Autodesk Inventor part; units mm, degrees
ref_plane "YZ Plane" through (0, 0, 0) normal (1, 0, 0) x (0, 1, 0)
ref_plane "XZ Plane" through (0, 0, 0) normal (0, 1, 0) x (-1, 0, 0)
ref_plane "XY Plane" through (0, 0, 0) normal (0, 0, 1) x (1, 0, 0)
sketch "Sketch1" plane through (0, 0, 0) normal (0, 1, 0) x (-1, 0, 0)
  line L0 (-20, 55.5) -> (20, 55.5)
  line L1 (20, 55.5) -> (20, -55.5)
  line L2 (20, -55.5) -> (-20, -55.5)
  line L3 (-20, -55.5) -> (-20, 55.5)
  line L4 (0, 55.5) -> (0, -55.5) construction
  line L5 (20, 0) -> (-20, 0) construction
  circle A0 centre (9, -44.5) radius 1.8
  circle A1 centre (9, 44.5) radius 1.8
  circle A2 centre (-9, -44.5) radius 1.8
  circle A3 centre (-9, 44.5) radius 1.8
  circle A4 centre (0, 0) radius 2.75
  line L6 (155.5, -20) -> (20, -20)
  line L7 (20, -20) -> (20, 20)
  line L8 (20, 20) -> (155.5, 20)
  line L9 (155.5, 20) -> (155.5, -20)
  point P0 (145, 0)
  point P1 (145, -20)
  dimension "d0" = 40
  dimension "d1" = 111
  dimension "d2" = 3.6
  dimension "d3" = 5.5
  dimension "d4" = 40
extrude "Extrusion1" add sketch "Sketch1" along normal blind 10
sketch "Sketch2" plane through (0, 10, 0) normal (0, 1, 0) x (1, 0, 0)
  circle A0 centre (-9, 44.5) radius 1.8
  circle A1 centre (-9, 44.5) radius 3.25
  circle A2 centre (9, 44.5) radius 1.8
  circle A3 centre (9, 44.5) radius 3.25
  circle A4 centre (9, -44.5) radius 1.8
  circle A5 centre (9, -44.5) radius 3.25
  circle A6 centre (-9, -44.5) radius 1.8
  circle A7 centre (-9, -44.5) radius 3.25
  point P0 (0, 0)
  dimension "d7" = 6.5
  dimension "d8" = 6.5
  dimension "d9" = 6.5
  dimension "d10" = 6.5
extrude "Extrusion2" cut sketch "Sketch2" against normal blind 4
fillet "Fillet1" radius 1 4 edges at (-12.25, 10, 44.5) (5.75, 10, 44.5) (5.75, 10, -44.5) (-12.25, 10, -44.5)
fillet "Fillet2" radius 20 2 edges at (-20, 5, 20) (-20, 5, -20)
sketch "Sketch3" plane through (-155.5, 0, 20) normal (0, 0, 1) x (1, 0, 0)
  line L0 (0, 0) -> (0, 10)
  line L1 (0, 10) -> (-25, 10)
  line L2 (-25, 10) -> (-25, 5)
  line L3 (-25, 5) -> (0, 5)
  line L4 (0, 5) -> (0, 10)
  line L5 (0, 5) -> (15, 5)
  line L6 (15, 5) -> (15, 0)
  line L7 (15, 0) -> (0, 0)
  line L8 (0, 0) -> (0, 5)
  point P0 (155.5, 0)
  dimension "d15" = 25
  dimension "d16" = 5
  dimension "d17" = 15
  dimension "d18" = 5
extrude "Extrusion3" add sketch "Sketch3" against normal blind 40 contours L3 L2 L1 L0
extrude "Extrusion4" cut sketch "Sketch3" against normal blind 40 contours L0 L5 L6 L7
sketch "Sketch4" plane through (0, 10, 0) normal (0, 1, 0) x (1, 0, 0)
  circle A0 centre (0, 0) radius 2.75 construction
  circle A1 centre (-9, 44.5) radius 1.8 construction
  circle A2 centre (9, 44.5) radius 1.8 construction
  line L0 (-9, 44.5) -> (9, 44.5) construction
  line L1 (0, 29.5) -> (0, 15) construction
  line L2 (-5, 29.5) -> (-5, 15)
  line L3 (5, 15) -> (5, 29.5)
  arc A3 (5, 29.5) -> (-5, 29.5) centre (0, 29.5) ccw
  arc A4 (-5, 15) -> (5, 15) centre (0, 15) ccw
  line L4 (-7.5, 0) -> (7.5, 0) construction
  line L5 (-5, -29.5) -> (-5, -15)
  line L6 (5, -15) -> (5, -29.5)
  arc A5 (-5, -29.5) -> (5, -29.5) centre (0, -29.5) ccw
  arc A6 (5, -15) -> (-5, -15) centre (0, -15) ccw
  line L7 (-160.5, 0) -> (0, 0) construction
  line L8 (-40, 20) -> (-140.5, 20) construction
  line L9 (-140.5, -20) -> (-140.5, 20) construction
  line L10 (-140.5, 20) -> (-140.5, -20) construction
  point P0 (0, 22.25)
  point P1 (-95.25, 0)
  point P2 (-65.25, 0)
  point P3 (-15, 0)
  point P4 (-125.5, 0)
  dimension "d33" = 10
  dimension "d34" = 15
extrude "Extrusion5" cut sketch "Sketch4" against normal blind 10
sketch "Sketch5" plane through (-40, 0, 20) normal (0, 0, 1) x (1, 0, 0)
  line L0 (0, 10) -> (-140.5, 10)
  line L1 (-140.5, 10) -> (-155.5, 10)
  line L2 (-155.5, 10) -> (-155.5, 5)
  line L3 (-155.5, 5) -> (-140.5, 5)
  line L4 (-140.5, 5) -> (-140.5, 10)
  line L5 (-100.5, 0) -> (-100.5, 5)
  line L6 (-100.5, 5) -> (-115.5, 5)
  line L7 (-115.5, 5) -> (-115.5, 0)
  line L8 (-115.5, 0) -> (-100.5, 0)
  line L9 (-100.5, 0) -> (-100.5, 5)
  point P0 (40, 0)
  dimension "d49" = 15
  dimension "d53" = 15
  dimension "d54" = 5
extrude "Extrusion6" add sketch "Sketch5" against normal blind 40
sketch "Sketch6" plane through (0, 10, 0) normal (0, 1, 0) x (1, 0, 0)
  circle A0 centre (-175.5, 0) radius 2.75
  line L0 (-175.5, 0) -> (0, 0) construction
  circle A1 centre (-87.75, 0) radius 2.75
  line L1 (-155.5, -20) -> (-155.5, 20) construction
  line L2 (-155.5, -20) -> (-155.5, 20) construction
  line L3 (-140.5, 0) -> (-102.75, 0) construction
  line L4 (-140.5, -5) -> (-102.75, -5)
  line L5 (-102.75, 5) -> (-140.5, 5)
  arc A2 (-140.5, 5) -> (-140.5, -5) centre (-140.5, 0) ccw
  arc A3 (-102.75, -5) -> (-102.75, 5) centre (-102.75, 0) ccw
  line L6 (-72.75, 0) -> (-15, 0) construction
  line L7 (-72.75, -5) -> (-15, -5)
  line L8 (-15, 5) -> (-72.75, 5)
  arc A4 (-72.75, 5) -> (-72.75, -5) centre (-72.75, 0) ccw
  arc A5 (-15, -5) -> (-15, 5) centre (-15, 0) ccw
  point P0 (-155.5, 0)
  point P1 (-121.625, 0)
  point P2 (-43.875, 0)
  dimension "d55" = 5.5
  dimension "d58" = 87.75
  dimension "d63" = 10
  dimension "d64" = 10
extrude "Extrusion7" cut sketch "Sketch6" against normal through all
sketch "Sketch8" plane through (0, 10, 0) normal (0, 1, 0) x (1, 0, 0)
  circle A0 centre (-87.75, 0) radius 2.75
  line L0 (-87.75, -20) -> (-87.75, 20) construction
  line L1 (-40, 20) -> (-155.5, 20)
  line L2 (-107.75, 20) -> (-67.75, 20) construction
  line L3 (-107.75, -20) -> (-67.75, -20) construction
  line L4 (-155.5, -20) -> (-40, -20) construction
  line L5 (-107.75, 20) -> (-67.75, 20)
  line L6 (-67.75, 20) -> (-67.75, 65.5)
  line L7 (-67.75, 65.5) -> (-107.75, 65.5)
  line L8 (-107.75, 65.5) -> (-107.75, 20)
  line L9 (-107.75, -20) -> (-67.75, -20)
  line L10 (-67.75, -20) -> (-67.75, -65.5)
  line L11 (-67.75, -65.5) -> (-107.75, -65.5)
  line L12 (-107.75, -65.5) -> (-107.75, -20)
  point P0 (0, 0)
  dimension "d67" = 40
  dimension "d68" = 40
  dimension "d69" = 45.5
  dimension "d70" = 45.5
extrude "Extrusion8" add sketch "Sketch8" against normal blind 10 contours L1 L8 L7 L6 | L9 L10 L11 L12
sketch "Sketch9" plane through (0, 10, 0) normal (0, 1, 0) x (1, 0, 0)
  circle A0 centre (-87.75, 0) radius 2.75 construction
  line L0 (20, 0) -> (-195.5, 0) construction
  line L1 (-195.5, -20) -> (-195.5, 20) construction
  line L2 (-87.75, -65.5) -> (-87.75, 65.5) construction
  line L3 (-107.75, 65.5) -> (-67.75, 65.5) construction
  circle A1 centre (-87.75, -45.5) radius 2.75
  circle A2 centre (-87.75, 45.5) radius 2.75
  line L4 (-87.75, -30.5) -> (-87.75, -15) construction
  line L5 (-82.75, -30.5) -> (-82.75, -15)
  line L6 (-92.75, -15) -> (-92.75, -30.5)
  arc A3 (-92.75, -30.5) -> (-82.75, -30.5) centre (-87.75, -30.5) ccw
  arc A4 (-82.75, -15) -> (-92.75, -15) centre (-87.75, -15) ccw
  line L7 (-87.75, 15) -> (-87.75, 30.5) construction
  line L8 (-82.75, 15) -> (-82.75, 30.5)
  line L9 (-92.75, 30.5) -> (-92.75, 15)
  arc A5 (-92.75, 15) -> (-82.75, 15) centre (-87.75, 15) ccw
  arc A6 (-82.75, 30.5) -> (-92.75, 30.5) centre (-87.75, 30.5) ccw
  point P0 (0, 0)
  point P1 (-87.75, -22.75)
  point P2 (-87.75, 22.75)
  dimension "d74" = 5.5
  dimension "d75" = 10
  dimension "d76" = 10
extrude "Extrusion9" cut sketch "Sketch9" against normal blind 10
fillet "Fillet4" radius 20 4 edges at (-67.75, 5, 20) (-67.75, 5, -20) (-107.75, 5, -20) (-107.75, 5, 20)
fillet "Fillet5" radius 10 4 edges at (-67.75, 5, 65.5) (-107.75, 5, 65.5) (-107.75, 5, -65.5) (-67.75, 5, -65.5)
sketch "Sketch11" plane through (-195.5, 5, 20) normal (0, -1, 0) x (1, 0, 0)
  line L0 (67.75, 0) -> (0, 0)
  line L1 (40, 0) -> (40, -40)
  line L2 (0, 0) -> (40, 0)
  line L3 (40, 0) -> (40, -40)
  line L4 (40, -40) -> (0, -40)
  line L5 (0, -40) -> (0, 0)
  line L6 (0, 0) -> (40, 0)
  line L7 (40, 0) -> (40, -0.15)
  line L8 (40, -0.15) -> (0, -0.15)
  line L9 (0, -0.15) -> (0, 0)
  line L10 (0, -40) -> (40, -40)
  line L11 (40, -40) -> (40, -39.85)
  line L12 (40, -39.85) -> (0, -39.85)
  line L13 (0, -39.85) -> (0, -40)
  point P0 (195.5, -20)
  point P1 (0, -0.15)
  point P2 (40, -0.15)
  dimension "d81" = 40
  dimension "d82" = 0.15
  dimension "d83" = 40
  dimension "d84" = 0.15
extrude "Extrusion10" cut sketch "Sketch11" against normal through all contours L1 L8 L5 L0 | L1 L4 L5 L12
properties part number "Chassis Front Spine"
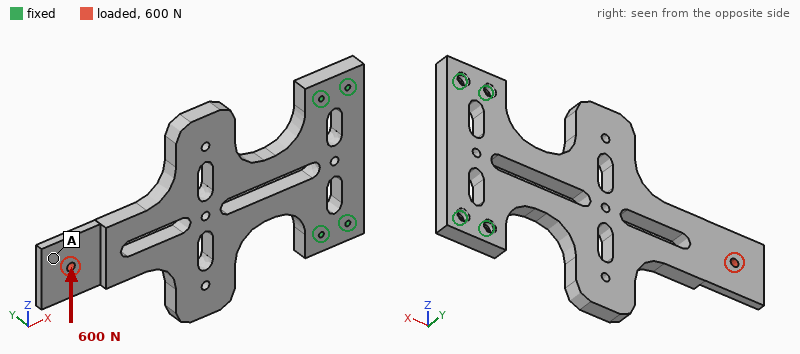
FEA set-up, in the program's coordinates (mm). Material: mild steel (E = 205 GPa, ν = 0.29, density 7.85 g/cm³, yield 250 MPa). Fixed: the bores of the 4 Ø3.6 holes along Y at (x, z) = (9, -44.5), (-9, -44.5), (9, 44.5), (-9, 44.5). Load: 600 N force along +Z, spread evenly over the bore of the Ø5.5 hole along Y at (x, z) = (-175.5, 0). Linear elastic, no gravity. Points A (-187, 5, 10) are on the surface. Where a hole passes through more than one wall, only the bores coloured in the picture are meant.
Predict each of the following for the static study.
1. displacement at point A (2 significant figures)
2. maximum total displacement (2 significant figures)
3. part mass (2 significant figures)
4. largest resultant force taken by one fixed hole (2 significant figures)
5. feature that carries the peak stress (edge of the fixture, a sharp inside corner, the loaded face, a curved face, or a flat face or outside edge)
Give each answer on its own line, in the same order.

0.098 mm
0.11 mm
980 g
750 N
a curved face
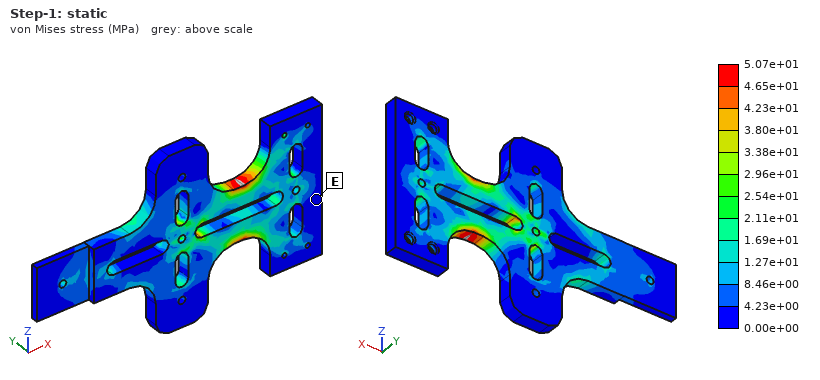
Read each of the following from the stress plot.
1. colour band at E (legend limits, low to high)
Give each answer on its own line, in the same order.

0.00e+00 to 4.23e+00 MPa
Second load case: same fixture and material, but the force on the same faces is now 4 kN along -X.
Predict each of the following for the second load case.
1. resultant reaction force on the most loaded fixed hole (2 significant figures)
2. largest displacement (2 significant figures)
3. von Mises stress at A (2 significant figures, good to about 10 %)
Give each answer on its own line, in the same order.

1.6 kN
0.30 mm
10 MPa
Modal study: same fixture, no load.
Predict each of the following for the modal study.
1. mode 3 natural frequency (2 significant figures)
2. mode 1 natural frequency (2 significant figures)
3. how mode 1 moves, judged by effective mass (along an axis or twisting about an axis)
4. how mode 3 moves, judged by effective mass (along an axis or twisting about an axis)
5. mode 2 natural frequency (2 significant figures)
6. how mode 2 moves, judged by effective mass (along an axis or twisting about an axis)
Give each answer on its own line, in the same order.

940 Hz
230 Hz
along Y
along Z
700 Hz
twisting about X
